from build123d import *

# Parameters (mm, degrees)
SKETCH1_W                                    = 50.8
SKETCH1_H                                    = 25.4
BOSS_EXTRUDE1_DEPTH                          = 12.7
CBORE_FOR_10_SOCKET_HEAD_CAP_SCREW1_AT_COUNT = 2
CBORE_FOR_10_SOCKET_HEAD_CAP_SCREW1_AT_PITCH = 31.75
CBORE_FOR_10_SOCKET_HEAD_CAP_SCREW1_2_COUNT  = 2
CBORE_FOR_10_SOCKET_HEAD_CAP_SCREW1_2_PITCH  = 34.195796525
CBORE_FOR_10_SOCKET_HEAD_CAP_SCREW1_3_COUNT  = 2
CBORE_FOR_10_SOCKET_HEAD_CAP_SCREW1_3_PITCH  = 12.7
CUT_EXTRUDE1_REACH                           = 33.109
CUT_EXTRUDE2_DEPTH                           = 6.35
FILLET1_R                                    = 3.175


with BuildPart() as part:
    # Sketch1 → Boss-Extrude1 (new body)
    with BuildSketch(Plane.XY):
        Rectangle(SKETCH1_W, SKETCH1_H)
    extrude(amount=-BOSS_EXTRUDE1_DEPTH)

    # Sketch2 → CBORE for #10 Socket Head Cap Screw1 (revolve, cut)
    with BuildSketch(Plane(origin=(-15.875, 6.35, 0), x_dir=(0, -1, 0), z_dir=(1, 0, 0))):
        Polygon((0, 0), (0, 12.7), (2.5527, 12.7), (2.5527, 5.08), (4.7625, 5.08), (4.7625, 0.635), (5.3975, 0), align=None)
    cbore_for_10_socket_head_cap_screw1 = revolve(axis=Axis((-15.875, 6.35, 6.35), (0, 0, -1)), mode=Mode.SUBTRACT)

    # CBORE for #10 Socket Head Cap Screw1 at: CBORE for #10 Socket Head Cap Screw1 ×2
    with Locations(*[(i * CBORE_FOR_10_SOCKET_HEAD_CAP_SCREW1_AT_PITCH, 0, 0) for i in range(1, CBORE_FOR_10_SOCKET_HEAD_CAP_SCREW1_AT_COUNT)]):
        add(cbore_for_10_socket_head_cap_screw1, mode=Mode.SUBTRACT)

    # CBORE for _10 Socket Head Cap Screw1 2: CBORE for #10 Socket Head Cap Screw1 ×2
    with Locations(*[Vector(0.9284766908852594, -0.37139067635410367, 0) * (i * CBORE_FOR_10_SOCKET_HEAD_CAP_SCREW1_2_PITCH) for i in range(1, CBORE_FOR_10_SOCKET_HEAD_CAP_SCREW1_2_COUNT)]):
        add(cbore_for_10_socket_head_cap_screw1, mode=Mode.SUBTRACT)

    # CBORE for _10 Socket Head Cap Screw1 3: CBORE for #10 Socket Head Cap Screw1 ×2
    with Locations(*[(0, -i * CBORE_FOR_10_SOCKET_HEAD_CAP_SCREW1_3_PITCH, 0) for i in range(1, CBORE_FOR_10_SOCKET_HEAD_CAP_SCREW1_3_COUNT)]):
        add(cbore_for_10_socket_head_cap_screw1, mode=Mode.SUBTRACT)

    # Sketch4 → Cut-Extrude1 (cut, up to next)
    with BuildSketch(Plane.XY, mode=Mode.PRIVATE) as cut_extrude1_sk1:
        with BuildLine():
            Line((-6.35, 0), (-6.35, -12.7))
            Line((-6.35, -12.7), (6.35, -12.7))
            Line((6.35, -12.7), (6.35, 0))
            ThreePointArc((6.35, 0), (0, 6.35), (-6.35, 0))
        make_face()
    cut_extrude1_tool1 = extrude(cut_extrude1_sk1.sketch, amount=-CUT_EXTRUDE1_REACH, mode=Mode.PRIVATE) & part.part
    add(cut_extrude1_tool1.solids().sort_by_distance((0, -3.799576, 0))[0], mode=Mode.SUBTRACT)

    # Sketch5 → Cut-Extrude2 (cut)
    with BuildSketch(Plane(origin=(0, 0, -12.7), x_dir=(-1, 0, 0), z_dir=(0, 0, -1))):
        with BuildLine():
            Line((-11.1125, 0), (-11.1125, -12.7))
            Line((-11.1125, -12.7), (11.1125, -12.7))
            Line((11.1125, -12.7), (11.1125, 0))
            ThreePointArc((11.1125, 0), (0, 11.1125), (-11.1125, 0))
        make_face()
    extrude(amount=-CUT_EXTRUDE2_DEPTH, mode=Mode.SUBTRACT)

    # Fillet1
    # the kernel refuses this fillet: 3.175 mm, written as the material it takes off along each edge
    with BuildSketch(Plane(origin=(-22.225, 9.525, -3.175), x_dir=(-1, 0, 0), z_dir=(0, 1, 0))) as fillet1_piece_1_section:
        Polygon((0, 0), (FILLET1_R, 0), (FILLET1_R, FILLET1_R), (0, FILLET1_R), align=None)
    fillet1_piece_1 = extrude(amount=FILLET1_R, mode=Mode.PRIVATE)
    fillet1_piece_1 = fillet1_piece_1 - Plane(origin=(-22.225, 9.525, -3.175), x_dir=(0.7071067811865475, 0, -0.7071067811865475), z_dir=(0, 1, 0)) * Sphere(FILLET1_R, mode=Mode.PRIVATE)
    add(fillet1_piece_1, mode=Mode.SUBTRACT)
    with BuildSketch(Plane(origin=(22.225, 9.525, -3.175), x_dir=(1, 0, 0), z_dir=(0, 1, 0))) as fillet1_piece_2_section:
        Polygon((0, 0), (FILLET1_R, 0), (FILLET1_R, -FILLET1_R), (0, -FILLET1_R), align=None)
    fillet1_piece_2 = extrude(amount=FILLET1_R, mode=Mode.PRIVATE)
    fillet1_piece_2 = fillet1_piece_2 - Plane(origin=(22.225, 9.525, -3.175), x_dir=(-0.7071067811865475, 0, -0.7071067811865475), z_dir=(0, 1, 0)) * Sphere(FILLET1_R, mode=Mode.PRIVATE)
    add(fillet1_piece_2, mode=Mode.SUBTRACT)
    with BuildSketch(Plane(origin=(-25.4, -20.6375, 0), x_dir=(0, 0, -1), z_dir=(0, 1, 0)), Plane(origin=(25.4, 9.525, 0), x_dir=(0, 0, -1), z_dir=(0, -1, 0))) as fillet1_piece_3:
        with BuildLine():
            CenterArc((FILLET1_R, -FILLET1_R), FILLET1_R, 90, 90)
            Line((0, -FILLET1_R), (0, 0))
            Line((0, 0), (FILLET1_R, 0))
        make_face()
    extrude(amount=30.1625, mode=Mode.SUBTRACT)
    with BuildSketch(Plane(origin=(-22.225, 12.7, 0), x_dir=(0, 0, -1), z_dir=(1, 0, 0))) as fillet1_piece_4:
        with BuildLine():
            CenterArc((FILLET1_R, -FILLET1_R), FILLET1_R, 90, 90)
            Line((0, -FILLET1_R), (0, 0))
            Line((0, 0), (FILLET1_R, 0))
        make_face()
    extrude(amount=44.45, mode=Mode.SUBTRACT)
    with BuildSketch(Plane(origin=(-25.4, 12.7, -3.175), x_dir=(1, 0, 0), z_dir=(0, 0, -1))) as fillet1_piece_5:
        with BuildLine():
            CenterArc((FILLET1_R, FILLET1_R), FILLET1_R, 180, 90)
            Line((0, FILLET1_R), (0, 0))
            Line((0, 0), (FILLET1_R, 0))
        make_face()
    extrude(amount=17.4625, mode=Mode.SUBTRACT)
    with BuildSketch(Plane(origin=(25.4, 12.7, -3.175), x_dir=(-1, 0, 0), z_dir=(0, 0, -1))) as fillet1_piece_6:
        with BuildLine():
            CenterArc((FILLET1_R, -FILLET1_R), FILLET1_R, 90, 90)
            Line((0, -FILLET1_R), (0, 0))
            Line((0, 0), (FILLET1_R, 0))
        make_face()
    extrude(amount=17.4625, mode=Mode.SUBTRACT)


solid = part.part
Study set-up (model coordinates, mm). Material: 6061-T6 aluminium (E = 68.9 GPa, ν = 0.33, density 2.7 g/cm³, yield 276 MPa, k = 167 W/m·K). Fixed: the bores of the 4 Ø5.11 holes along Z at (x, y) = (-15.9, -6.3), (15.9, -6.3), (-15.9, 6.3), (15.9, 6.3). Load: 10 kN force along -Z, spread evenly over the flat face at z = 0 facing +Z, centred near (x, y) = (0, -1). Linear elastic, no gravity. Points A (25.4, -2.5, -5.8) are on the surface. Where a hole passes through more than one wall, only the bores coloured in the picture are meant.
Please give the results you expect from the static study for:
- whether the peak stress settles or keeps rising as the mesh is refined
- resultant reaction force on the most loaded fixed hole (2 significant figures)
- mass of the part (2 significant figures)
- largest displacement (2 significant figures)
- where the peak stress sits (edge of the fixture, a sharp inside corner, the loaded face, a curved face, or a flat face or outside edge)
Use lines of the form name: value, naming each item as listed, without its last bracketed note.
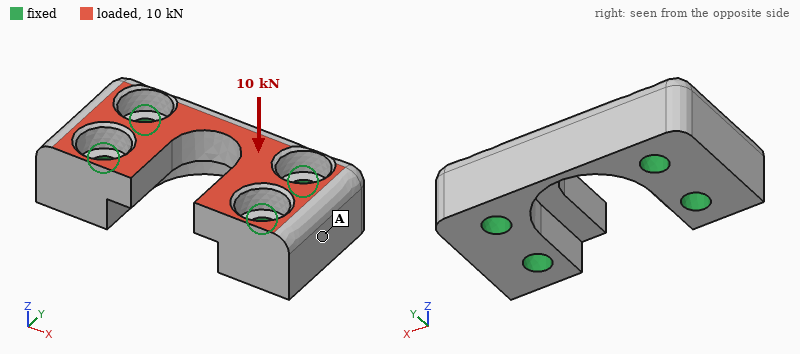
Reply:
whether the peak stress settles or keeps rising as the mesh is refined: keeps rising
resultant reaction force on the most loaded fixed hole: 2.8 kN
mass of the part: 26 g
largest displacement: 29 µm
where the peak stress sits: edge of the fixture
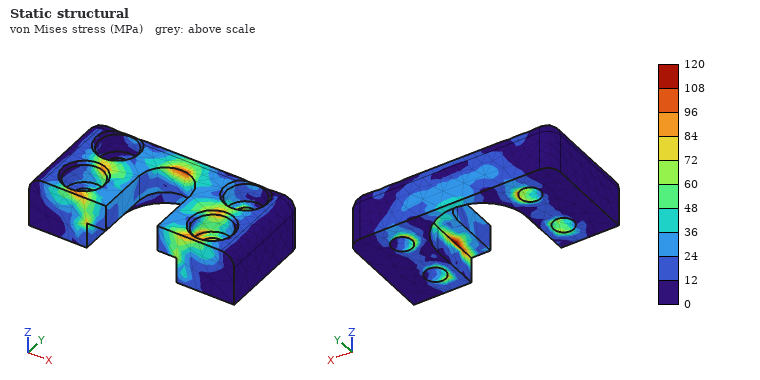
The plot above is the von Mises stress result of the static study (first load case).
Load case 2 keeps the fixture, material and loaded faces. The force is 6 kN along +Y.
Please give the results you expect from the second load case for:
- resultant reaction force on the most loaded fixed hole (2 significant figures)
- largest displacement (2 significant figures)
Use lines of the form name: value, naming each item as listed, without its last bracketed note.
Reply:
resultant reaction force on the most loaded fixed hole: 2.1 kN
largest displacement: 17 µm
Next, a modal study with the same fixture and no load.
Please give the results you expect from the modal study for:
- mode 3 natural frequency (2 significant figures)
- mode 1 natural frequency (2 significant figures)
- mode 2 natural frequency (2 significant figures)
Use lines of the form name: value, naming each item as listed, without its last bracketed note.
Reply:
mode 3 natural frequency: 40 kHz
mode 1 natural frequency: 35 kHz
mode 2 natural frequency: 37 kHz
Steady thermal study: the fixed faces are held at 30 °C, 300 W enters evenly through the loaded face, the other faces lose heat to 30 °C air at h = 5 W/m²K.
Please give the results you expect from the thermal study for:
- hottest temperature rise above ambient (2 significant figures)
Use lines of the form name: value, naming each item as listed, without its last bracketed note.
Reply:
hottest temperature rise above ambient: 51 K
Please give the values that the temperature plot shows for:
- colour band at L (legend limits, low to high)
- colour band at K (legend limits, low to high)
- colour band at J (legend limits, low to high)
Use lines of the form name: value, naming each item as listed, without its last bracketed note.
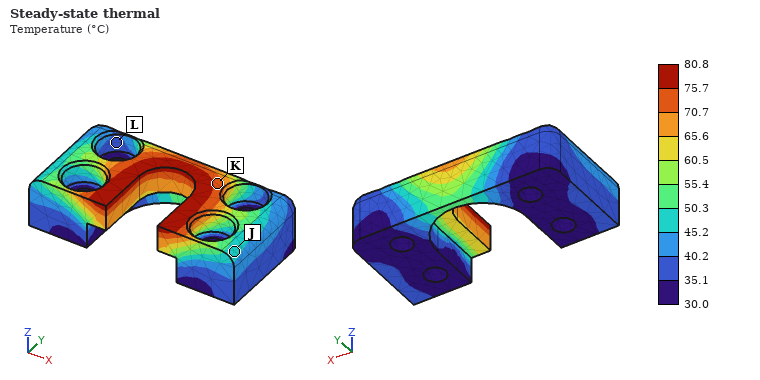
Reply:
colour band at L: 35.1 to 40.2 °C
colour band at K: 70.7 to 75.7 °C
colour band at J: 45.2 to 50.3 °C
